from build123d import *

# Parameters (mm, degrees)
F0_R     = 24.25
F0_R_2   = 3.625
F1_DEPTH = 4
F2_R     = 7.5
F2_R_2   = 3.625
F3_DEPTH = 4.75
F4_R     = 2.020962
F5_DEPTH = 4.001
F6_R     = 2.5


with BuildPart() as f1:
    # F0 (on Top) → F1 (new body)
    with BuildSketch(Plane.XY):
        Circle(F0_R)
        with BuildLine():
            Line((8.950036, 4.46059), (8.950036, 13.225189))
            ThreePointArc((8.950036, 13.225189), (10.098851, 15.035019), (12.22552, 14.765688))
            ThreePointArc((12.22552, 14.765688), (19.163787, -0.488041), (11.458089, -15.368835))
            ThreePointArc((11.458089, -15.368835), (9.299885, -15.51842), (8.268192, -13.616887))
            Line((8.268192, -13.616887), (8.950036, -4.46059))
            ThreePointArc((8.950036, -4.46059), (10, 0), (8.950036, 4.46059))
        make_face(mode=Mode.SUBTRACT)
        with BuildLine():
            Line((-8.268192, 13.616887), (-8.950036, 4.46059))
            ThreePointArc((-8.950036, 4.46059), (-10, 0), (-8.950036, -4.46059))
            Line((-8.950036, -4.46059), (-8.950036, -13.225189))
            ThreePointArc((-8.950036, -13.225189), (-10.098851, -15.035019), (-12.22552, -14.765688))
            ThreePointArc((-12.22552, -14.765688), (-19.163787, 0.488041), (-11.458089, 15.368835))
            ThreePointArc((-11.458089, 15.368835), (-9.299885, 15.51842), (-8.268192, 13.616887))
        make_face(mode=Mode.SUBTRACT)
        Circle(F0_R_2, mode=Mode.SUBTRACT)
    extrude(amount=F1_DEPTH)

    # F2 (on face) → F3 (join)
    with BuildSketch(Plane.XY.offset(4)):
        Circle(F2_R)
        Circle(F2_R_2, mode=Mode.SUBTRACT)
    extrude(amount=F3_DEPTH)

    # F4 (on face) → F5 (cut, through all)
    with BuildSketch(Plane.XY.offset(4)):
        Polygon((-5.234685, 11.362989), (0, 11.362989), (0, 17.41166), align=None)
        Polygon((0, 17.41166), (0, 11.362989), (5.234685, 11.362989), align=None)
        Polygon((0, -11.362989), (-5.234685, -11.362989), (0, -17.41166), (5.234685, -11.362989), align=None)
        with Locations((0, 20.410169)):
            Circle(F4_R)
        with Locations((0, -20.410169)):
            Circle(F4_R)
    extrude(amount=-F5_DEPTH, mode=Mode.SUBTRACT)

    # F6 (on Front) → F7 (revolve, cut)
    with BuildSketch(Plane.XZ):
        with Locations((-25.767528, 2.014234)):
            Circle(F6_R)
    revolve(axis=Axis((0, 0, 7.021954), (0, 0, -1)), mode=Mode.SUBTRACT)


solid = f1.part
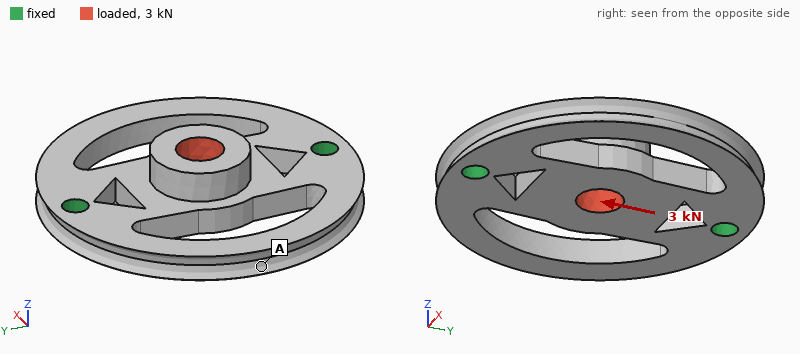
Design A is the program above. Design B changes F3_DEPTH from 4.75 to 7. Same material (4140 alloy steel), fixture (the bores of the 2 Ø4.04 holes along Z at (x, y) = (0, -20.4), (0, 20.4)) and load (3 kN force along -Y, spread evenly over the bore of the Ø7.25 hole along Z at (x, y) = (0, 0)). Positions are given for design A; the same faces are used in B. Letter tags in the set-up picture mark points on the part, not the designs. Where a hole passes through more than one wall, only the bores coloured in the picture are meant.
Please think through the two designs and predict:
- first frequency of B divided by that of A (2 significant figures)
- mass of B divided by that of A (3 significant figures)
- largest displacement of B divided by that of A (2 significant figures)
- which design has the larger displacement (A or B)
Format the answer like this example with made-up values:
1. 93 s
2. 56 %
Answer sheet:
1. 0.99
2. 1.06
3. 1.4
4. B
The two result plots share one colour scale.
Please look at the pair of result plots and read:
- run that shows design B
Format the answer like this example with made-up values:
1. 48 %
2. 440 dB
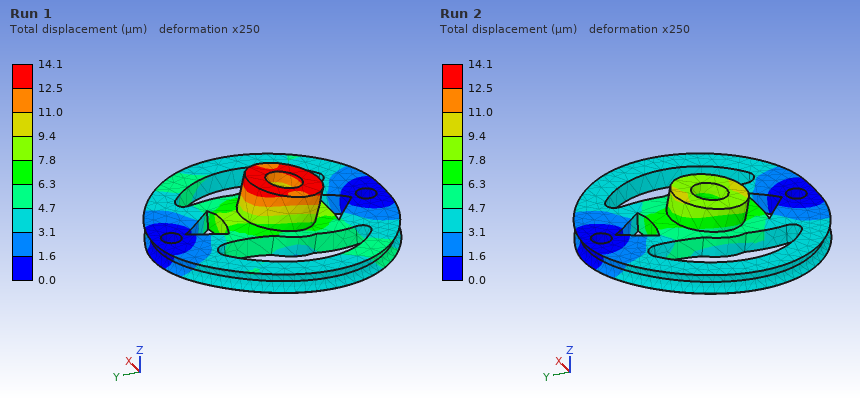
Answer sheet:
1. Run 1
